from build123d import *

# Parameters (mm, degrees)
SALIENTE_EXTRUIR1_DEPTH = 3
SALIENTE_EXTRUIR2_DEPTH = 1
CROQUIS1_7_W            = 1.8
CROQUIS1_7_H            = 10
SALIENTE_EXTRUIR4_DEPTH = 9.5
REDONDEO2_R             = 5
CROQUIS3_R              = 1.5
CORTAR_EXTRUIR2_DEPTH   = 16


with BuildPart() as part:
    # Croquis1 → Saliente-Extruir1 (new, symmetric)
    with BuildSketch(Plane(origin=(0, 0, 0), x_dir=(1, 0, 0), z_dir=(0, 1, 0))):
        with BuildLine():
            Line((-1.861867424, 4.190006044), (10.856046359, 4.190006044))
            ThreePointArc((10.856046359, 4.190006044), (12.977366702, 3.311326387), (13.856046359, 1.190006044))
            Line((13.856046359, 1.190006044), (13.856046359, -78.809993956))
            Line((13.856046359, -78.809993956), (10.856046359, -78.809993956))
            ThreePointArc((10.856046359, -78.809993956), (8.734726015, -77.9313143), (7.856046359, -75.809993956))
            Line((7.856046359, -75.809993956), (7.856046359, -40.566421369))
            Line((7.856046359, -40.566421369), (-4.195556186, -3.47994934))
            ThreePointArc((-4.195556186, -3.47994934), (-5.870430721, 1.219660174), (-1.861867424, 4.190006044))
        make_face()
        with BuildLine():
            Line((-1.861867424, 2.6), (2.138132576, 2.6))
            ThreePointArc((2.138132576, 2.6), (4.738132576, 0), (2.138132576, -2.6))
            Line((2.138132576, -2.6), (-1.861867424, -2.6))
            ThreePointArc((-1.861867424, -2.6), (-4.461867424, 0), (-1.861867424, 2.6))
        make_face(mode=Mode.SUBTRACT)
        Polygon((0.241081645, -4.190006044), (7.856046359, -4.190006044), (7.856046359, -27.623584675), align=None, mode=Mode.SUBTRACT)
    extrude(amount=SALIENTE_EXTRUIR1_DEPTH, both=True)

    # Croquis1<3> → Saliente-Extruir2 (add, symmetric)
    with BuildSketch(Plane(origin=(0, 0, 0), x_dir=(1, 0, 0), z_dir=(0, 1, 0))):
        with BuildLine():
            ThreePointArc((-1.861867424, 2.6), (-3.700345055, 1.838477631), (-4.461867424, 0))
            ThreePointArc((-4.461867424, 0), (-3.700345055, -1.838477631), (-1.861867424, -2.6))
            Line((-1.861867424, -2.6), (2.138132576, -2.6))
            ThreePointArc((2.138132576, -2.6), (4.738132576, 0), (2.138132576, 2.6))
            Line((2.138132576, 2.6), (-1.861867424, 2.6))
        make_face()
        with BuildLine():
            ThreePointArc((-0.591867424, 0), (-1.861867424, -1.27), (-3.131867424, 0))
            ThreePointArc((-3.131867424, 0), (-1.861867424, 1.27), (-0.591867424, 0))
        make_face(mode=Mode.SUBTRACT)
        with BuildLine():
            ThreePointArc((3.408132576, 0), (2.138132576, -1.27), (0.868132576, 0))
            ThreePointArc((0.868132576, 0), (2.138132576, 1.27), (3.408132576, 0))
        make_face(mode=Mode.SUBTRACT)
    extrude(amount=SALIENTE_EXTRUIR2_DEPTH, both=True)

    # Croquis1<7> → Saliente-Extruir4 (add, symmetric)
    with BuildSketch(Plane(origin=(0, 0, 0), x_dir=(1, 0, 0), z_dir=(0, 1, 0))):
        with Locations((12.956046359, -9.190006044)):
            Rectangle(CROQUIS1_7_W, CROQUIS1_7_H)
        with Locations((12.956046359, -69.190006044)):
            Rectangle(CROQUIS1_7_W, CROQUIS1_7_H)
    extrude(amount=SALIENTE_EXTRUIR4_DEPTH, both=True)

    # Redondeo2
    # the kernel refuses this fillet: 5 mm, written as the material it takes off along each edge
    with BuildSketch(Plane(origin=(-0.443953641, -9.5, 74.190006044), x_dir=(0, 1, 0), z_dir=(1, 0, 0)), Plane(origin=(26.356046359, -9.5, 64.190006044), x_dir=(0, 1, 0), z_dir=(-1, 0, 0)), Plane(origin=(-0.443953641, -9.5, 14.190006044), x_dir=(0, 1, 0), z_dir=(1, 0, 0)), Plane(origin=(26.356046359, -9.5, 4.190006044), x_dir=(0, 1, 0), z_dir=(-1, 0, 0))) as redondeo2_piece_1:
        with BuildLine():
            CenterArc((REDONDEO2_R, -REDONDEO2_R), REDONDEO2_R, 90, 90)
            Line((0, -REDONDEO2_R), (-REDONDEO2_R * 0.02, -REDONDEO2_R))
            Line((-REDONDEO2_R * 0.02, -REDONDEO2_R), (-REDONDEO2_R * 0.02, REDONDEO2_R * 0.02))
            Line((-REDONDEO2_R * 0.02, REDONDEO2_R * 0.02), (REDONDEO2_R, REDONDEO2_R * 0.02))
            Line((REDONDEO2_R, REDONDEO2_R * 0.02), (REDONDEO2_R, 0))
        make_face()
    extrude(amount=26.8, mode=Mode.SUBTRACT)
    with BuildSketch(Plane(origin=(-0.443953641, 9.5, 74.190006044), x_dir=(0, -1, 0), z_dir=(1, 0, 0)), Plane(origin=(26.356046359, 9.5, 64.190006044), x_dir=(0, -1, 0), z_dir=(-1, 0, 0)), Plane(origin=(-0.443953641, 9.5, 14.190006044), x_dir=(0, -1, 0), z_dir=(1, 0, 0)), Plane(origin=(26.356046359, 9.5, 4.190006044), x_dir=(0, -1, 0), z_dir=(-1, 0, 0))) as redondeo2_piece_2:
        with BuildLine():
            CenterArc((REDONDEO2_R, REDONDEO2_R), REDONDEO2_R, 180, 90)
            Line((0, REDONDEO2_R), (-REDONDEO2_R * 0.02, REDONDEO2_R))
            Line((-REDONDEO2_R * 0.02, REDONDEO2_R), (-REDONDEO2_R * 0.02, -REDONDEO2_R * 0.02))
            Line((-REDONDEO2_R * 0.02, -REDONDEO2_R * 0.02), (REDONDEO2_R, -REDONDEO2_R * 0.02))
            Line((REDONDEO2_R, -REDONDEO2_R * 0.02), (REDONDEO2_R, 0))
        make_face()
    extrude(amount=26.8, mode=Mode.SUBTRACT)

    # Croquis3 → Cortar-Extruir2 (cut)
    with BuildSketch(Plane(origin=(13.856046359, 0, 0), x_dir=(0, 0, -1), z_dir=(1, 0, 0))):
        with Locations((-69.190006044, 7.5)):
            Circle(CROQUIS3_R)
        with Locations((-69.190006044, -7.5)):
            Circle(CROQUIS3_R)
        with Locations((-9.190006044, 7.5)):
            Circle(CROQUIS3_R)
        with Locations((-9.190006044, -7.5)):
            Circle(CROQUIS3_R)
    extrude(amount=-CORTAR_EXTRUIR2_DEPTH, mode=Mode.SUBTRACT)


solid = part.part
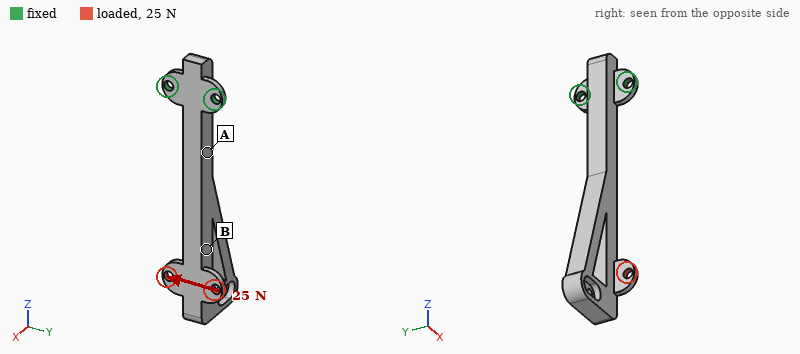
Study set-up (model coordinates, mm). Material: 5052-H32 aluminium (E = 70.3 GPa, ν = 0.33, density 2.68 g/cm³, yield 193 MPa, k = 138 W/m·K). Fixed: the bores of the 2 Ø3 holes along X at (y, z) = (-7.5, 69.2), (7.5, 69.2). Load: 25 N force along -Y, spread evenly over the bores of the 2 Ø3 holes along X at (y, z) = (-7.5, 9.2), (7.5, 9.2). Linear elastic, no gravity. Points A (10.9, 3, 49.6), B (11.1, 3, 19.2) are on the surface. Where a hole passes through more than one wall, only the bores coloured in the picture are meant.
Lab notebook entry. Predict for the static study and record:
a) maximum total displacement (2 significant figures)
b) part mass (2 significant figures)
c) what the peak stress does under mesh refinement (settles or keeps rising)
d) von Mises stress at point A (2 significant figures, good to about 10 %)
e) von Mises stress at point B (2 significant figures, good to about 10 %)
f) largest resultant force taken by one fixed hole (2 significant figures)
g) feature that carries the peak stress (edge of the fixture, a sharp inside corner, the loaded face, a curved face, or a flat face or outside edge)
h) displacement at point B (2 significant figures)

0.29 mm
12 g
keeps rising
28 MPa
5.6 MPa
100 N
a sharp inside corner
0.17 mm
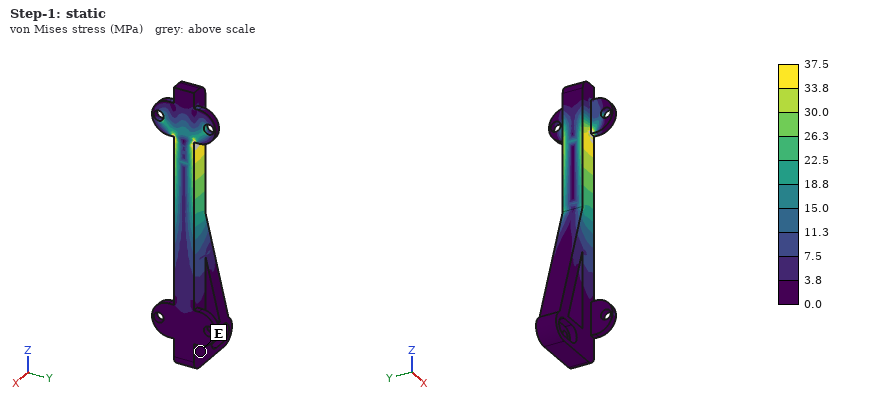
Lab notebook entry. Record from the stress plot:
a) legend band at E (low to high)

0.0 to 3.8 MPa
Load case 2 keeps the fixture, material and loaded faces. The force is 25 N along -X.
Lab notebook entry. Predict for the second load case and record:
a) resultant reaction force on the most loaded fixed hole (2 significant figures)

48 N
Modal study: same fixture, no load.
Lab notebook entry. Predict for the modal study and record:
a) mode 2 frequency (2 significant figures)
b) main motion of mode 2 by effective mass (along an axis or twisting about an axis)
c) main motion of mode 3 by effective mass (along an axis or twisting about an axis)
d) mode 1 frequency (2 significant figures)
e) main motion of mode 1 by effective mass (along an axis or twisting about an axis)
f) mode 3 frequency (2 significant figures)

650 Hz
along Y
twisting about Z
430 Hz
along X
3500 Hz
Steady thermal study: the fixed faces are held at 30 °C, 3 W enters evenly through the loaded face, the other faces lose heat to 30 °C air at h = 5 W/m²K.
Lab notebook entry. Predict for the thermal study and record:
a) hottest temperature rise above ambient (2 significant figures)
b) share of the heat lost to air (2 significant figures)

36 K
12 %
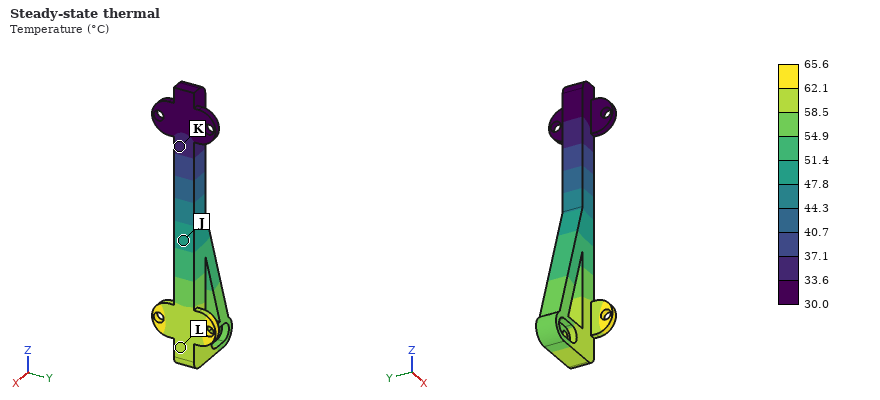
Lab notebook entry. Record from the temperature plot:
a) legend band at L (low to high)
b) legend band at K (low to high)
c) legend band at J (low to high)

58.5 to 62.1 °C
33.6 to 37.1 °C
47.8 to 51.4 °C
